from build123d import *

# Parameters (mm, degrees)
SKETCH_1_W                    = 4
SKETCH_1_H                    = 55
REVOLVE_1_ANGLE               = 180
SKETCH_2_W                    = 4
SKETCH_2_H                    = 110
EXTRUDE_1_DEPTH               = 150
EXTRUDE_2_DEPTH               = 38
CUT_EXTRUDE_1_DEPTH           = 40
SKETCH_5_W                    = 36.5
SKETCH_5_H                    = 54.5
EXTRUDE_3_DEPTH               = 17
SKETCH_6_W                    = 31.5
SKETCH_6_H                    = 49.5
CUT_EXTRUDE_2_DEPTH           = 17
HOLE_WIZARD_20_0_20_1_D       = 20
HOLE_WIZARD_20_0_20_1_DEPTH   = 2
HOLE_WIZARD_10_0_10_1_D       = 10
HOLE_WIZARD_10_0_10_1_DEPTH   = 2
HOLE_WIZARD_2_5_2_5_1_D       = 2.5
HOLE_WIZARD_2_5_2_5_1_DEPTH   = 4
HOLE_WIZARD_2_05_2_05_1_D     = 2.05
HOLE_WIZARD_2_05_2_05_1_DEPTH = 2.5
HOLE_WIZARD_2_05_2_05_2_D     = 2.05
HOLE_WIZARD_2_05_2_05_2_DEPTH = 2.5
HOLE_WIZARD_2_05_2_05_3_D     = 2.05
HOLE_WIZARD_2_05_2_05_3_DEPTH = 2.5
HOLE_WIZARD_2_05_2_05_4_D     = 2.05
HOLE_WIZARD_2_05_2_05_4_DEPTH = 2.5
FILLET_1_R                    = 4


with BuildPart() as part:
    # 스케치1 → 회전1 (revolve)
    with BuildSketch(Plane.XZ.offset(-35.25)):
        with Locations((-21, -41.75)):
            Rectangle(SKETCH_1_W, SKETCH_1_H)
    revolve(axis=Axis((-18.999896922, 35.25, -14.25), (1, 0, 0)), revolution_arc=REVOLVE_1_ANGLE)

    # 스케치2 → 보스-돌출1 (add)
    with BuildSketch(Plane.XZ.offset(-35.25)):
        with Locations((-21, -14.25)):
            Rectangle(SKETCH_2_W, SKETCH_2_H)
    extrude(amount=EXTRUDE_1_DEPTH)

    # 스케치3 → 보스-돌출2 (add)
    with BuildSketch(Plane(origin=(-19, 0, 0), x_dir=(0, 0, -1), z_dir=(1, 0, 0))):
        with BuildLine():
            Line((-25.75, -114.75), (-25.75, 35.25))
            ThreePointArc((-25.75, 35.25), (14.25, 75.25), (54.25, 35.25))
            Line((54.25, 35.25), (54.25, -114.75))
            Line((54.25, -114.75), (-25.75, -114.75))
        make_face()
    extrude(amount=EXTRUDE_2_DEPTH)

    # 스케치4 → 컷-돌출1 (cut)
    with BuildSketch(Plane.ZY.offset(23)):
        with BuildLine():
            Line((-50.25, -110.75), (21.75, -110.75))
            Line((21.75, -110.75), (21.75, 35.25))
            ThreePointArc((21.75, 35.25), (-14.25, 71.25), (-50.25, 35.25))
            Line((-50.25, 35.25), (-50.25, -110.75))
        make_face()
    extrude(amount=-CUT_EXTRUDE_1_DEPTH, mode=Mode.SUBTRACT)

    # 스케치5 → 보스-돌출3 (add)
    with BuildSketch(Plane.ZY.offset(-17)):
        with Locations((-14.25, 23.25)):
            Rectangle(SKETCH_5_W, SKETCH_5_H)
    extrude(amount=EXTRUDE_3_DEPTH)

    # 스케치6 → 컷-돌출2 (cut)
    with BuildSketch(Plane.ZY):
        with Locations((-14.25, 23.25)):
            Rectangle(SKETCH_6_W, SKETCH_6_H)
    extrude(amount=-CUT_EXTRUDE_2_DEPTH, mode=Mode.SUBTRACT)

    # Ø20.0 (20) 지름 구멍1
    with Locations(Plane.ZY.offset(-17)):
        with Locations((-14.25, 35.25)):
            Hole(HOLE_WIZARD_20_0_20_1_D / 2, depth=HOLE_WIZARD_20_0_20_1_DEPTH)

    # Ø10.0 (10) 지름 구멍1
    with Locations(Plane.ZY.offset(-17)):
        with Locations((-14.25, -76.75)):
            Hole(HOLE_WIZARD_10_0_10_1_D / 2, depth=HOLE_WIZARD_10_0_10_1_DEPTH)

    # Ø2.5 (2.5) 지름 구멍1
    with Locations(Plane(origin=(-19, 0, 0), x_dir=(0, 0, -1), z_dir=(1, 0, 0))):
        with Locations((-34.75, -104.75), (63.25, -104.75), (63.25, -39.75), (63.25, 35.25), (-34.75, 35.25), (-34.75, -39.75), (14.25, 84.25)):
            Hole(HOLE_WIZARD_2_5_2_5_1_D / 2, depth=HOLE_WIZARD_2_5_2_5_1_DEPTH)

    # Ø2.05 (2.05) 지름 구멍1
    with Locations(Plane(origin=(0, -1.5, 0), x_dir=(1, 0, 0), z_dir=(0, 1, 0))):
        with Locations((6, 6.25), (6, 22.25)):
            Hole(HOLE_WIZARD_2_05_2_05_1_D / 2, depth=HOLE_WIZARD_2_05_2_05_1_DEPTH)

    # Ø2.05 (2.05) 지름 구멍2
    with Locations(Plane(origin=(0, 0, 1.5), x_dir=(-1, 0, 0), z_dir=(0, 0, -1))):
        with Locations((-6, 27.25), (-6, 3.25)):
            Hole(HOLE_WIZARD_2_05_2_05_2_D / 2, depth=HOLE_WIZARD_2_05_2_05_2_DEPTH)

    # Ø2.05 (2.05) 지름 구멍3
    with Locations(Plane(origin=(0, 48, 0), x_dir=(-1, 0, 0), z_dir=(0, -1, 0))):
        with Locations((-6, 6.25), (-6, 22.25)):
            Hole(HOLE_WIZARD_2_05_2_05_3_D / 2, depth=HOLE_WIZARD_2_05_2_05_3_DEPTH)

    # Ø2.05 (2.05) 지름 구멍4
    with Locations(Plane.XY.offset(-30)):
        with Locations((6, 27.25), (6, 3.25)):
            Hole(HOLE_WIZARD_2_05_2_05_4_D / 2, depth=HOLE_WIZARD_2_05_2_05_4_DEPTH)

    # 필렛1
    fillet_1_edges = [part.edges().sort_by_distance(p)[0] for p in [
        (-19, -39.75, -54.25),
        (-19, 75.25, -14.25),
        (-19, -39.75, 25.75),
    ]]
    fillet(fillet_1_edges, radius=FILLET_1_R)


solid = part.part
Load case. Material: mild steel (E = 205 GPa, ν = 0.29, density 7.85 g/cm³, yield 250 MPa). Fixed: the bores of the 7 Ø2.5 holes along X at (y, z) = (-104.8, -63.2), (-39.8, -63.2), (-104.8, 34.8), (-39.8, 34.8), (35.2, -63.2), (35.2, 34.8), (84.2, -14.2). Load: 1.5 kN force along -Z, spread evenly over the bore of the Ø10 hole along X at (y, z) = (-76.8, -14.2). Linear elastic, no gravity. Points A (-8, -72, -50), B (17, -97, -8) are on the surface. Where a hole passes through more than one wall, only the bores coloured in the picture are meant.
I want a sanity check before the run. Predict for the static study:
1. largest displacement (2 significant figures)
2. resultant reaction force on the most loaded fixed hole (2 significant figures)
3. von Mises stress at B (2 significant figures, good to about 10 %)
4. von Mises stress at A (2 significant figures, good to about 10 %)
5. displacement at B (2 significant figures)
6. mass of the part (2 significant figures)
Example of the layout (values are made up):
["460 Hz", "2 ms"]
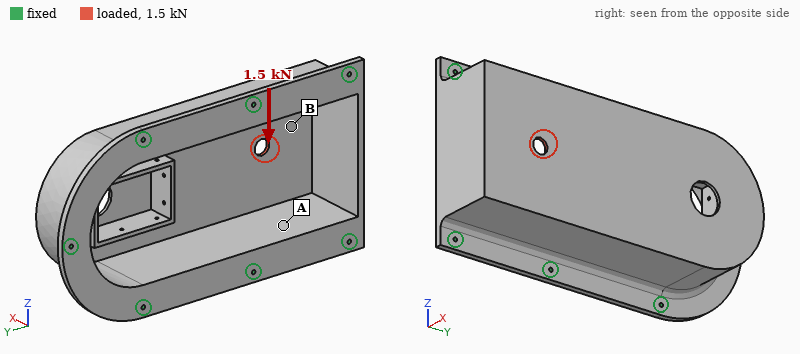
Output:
["12 µm", "700 N", "14 MPa", "4.2 MPa", "8.1 µm", "1.1 kg"]
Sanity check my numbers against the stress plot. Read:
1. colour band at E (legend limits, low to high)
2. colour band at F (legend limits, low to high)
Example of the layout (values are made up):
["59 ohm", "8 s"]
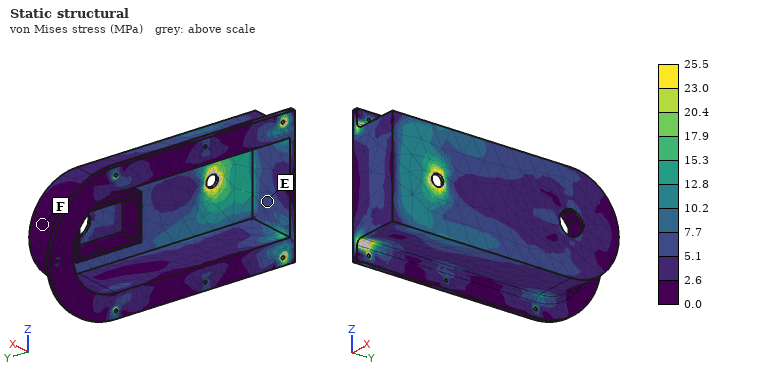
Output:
["5.1 to 7.7 MPa", "0.0 to 2.6 MPa"]
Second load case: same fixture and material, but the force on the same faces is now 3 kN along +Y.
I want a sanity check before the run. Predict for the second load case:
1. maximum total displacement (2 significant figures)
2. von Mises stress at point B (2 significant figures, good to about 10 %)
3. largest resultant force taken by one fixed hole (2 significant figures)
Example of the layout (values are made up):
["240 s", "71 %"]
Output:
["10.0 µm", "16 MPa", "570 N"]
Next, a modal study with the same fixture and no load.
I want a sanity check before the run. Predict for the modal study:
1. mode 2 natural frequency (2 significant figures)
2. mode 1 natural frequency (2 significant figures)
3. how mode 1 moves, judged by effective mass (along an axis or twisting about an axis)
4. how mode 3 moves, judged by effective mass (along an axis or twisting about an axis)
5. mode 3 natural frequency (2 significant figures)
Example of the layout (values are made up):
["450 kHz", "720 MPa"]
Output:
["2700 Hz", "2300 Hz", "along X", "along Z", "3000 Hz"]
